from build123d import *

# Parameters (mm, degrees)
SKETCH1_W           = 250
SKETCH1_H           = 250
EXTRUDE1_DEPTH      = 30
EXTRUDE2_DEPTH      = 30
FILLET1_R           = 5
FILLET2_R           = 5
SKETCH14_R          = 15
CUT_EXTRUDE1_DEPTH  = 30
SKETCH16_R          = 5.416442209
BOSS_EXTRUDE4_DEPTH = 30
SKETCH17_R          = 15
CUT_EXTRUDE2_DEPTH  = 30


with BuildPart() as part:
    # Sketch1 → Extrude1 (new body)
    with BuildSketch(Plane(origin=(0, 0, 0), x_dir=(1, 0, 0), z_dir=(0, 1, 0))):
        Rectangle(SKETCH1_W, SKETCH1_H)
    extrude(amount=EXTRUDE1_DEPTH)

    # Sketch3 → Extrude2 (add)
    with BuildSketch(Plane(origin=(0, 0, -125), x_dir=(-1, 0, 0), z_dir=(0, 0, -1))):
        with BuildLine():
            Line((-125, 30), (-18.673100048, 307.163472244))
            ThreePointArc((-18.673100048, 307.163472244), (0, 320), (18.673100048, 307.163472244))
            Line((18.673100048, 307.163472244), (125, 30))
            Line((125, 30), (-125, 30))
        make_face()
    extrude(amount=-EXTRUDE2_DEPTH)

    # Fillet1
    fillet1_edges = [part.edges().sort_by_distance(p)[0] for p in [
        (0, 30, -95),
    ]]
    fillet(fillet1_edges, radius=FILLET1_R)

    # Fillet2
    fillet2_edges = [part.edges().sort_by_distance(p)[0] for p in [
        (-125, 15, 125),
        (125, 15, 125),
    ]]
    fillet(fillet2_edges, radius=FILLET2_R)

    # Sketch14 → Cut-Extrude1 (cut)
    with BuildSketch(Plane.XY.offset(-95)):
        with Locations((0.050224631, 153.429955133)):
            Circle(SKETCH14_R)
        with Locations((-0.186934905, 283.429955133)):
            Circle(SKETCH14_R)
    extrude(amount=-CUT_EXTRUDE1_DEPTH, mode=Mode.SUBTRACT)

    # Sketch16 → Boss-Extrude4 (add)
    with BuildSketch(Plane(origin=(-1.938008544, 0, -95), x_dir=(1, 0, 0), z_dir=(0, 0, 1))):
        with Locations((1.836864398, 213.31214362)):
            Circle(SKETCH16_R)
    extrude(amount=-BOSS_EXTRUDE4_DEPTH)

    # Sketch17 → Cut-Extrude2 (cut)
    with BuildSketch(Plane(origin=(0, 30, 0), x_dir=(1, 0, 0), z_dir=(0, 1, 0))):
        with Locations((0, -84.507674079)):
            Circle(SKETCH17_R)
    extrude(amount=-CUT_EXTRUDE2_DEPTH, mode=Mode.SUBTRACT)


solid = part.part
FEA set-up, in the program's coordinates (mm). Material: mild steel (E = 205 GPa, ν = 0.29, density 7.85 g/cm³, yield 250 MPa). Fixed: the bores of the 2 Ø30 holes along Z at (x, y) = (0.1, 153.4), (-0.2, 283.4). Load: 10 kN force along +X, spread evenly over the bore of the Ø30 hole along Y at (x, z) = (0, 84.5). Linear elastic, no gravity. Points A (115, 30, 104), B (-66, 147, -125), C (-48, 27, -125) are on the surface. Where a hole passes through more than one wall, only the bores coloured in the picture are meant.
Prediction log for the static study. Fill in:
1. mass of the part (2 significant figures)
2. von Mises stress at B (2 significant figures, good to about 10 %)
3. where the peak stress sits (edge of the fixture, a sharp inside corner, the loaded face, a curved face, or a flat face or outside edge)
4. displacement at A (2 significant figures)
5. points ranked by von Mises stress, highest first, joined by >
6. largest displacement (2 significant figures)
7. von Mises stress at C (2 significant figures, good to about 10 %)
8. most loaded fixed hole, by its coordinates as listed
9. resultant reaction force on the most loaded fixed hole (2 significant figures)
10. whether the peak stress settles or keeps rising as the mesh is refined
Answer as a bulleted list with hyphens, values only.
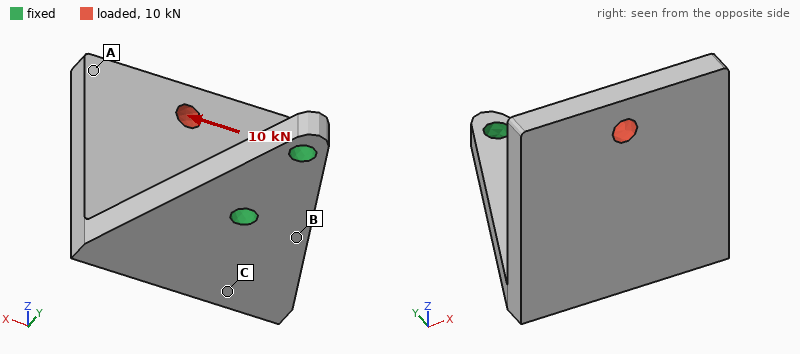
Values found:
- 24 kg
- 47 MPa
- edge of the fixture
- 0.46 mm
- B > C > A
- 0.49 mm
- 27 MPa
- (0.1, 153.4)
- 17 kN
- keeps rising
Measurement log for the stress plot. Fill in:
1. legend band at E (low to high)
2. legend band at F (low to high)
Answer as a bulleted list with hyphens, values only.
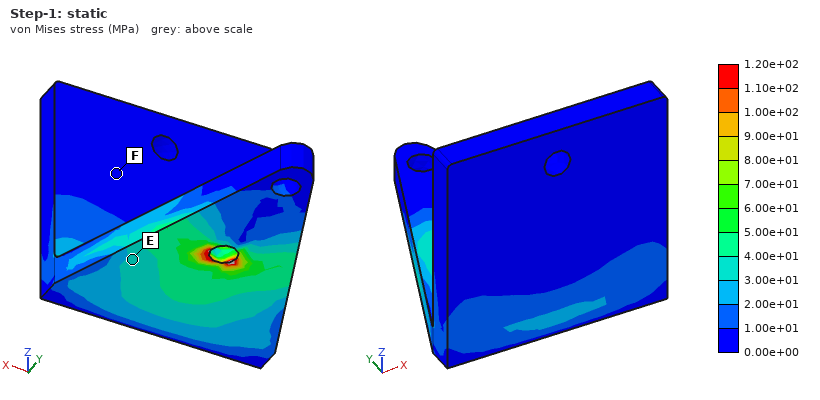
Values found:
- 3.00e+01 to 4.00e+01 MPa
- 0.00e+00 to 1.00e+01 MPa
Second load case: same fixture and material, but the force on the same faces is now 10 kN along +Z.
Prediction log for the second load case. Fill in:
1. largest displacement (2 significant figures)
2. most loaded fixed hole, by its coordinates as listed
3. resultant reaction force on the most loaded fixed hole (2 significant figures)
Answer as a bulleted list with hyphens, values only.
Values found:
- 0.30 mm
- (0.1, 153.4)
- 12 kN
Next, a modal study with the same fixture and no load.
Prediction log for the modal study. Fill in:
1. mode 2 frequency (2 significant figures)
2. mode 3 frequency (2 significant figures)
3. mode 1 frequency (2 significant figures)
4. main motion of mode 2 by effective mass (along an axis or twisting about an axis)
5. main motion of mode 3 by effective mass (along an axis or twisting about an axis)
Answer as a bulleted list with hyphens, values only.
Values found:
- 280 Hz
- 640 Hz
- 210 Hz
- along X
- along Z
